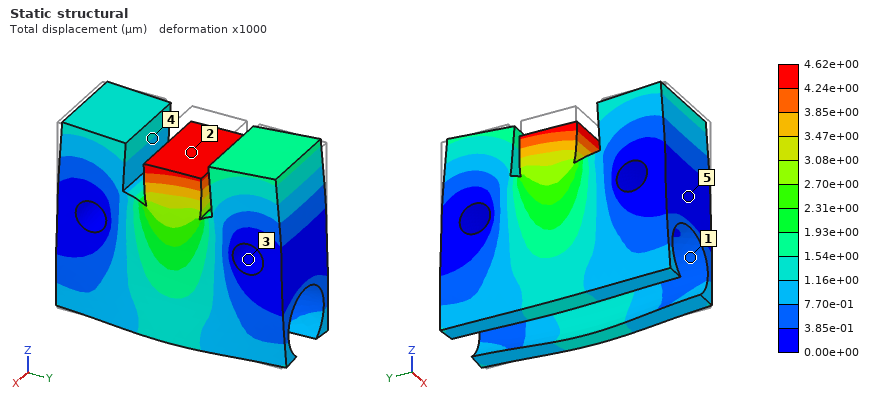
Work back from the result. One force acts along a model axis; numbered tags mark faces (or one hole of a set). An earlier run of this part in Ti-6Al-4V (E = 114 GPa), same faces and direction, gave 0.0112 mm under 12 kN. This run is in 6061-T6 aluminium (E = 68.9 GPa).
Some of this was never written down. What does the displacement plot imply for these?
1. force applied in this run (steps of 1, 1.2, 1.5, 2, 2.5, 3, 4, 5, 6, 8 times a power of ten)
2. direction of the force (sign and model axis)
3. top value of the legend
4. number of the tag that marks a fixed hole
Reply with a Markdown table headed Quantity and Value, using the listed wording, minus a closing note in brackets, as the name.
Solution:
| Quantity | Value |
|---|---|
| force applied in this run | 3 kN |
| direction of the force | -Z |
| top value of the legend | 4.62e+00 µm |
| number of the tag that marks a fixed hole | 3 |
